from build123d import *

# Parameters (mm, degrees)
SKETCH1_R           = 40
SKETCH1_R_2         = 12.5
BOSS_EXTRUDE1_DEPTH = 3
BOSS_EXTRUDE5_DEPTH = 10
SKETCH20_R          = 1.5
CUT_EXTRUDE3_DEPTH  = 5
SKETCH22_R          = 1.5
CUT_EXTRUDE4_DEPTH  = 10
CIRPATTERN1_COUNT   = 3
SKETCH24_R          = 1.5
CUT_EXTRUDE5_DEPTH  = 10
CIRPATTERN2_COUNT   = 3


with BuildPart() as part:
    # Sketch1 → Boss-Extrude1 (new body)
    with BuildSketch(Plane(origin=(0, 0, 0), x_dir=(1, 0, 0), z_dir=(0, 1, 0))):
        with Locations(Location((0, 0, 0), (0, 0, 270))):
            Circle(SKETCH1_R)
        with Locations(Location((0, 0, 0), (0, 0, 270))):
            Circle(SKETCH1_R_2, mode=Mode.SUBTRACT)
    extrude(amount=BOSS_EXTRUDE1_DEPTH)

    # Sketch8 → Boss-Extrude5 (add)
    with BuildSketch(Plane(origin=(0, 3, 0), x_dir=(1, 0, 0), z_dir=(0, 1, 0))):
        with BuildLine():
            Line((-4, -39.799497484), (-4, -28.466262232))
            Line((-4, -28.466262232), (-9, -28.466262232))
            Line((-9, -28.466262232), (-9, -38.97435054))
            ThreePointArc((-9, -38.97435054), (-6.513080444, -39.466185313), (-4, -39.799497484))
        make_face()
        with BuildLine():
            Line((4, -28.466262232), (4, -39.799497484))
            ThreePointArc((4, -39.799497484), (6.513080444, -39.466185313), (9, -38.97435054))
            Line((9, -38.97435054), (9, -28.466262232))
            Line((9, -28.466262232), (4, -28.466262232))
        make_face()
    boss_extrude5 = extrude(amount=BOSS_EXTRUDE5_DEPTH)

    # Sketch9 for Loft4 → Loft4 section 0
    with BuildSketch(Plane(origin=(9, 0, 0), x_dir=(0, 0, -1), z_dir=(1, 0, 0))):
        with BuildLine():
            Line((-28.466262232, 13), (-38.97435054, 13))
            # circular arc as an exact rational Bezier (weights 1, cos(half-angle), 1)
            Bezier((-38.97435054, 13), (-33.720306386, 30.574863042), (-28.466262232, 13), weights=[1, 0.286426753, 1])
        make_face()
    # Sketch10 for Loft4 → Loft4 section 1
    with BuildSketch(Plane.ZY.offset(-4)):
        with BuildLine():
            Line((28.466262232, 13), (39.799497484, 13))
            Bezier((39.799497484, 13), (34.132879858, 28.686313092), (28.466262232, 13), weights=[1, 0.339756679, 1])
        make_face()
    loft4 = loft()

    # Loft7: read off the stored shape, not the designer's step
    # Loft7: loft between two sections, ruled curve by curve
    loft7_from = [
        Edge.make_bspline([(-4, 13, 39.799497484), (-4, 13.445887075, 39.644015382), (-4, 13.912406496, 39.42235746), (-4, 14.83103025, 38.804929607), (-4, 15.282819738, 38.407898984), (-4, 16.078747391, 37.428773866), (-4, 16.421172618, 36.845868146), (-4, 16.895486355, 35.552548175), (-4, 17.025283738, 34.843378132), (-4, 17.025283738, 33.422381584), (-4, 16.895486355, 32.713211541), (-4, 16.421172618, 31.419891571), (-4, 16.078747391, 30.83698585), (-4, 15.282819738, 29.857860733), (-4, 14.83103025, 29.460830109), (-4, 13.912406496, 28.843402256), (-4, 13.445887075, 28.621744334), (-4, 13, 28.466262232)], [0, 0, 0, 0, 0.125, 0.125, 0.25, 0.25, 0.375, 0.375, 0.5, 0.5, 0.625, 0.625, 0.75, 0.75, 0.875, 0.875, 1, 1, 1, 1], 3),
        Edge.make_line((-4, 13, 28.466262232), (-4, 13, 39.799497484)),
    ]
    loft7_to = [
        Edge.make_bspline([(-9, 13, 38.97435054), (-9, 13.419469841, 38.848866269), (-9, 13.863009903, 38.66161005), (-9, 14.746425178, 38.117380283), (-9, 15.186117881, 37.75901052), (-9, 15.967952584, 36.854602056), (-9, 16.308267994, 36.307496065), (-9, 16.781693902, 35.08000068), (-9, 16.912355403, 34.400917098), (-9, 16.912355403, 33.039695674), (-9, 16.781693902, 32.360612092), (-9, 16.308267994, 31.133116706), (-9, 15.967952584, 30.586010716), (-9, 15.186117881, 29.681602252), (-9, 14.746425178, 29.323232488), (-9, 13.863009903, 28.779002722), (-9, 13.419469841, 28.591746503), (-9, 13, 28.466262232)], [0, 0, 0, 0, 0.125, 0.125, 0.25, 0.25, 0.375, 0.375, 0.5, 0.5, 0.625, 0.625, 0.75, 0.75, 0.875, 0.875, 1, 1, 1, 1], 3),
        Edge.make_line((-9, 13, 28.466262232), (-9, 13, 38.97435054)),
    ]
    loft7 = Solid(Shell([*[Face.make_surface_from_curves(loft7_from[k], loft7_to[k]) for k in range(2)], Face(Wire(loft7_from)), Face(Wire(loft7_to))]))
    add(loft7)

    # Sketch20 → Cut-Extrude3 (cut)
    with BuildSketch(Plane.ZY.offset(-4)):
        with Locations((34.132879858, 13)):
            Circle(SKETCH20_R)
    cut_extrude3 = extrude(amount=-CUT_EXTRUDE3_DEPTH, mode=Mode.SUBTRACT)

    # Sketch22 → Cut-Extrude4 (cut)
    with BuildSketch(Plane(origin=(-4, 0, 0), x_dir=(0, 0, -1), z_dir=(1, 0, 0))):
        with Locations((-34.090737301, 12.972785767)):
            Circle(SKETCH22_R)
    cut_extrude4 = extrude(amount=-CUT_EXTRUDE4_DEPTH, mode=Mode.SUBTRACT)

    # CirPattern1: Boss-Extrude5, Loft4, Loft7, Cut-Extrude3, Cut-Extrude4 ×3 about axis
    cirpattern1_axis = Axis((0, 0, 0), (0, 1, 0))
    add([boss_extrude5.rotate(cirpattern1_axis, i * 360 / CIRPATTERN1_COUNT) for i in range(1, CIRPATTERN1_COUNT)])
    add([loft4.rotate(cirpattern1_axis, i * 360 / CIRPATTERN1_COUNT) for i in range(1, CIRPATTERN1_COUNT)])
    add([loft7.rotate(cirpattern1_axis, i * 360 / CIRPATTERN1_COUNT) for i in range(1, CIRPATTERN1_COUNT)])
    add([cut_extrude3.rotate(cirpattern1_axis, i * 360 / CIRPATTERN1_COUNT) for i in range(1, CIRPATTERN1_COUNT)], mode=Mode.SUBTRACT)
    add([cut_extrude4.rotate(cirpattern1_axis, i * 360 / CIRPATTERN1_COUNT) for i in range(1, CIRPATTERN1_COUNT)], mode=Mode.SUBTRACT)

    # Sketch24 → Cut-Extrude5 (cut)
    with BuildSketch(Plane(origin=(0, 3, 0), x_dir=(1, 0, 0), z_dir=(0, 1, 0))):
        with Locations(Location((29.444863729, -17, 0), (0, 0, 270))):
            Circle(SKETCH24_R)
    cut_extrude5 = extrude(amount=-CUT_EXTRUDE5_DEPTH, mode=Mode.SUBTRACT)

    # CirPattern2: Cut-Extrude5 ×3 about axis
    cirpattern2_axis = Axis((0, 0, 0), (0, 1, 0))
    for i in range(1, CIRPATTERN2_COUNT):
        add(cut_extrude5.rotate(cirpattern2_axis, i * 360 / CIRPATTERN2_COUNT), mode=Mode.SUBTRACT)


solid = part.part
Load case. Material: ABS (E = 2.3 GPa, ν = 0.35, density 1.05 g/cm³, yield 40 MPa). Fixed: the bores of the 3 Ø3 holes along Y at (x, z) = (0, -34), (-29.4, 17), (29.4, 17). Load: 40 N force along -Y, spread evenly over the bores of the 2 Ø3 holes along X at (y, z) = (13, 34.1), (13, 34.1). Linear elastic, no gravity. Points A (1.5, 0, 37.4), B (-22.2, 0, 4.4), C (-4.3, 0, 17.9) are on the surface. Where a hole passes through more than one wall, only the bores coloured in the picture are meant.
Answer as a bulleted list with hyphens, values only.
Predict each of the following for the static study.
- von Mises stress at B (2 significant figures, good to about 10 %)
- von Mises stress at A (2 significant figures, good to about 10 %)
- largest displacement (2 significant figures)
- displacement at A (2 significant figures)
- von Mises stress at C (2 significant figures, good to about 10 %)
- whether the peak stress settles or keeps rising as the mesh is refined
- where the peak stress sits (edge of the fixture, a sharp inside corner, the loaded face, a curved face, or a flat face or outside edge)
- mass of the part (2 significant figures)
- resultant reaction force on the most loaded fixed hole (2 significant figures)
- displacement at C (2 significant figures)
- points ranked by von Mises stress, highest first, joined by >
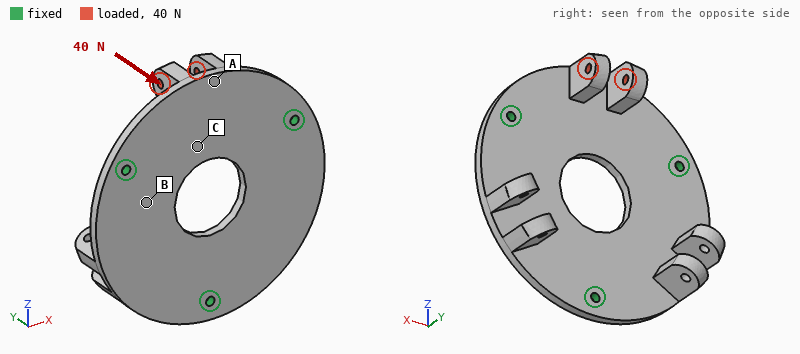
- 1.9 MPa
- 6.8 MPa
- 1.2 mm
- 0.99 mm
- 4.6 MPa
- keeps rising
- edge of the fixture
- 18 g
- 22 N
- 0.28 mm
- A > C > B
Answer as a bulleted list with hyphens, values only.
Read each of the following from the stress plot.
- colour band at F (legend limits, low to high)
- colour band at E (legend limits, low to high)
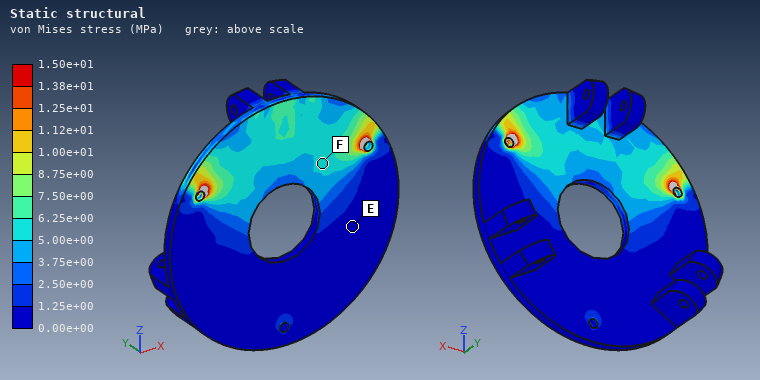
- 5.00e+00 to 6.25e+00 MPa
- 0.00e+00 to 1.25e+00 MPa
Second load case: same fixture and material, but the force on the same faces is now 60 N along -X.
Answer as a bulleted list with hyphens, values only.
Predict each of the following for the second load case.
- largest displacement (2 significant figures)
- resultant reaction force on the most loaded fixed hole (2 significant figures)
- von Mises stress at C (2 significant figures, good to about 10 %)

- 0.39 mm
- 38 N
- 2.2 MPa
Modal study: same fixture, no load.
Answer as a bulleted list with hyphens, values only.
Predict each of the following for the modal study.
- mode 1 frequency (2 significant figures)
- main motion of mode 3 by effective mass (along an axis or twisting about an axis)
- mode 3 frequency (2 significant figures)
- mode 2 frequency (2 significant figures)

- 600 Hz
- along Y
- 700 Hz
- 600 Hz
